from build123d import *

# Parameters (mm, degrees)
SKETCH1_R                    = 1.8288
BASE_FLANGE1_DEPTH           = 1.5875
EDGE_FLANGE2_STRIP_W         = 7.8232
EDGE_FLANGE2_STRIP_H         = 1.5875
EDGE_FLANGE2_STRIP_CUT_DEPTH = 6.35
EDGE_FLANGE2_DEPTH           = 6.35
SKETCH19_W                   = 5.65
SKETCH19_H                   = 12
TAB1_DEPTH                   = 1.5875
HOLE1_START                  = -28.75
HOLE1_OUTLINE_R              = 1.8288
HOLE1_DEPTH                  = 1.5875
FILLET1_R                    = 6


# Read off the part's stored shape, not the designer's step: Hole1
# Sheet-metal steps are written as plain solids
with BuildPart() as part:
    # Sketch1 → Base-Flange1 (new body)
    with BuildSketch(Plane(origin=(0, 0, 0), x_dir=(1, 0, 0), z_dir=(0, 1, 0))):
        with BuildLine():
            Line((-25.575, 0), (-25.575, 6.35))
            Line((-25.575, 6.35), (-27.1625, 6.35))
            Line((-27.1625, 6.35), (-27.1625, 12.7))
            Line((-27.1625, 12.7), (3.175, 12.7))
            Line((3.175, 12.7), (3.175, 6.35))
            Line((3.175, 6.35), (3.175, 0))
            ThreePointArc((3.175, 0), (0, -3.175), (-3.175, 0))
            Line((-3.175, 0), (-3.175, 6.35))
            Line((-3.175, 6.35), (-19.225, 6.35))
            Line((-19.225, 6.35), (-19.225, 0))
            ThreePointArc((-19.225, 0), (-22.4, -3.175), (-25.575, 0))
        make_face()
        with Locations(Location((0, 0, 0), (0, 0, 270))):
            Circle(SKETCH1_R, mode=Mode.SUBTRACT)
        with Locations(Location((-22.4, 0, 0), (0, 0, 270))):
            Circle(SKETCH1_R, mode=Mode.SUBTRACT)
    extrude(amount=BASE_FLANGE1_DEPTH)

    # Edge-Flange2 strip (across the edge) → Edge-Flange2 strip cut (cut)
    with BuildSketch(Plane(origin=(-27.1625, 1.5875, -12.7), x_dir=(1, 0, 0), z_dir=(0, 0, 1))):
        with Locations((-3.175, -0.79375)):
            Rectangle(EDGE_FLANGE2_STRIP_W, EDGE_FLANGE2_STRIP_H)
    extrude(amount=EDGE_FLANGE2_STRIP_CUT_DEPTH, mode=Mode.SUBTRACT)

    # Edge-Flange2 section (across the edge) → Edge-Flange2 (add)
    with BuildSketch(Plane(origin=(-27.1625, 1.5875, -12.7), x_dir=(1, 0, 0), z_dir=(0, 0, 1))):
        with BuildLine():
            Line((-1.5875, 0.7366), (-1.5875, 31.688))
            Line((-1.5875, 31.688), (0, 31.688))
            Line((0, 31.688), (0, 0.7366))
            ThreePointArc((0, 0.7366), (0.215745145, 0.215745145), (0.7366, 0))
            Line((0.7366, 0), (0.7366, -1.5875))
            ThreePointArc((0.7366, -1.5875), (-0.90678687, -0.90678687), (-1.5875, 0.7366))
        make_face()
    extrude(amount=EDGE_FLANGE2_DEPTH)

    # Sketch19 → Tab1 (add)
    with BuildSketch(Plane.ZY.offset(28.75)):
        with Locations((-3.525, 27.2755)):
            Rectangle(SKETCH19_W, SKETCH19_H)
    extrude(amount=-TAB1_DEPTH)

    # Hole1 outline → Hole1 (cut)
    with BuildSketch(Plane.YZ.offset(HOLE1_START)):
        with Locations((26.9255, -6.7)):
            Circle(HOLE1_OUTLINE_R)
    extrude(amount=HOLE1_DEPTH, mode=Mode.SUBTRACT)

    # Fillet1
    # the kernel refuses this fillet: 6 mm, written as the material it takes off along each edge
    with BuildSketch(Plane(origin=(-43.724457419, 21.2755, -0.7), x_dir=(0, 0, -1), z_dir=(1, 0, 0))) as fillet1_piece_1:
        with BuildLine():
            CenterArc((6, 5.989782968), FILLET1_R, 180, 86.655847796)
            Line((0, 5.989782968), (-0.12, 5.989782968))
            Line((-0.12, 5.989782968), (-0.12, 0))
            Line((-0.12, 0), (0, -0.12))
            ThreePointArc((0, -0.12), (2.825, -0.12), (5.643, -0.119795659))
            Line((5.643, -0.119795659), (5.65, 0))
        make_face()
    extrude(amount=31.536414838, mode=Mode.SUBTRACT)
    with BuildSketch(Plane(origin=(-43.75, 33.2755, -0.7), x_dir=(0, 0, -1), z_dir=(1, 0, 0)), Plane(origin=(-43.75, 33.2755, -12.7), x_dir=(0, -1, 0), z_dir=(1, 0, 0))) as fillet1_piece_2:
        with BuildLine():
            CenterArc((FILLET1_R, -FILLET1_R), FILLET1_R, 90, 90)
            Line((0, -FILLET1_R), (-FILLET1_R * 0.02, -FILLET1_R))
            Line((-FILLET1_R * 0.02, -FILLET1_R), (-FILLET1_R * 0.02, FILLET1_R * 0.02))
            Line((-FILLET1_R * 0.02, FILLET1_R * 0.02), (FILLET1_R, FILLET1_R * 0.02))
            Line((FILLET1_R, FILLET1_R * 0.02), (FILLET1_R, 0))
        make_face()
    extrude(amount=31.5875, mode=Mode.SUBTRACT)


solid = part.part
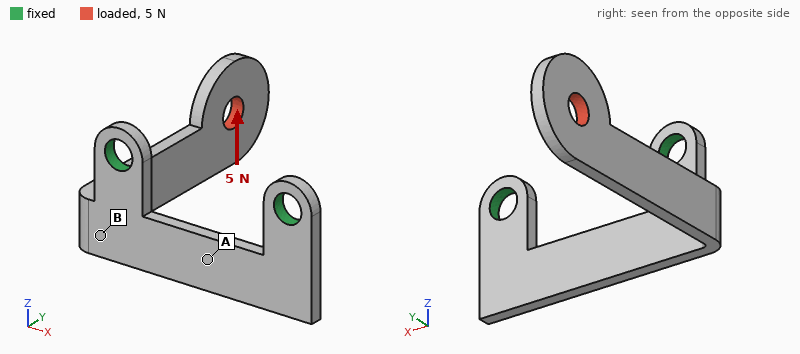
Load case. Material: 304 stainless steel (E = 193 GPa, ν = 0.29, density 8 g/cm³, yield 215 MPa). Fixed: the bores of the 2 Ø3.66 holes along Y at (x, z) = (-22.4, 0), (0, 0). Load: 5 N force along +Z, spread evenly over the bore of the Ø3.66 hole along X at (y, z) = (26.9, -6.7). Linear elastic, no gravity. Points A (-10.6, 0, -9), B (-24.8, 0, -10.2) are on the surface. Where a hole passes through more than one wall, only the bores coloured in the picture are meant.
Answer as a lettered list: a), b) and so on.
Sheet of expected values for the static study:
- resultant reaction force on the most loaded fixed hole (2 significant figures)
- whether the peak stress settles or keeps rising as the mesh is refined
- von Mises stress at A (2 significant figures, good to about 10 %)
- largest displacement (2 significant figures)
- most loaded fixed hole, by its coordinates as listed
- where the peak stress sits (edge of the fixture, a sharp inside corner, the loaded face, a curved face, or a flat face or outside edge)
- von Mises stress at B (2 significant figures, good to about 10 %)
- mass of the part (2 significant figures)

a) 6.0 N
b) keeps rising
c) 11 MPa
d) 87 µm
e) (-22.4, 0)
f) a sharp inside corner
g) 31 MPa
h) 6.7 g
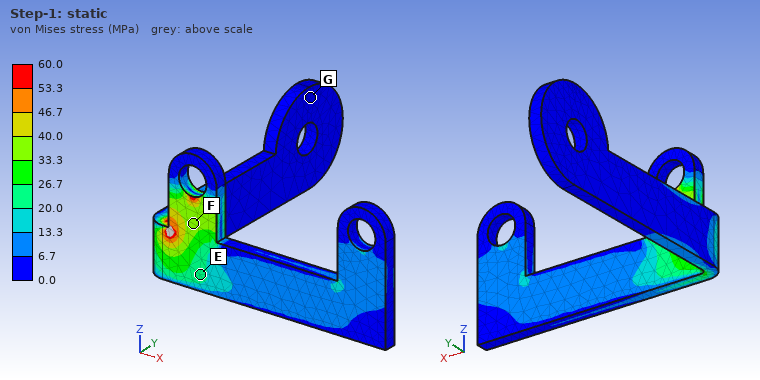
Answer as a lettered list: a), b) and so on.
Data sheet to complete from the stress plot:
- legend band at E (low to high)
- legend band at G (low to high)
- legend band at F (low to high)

a) 20.0 to 26.7 MPa
b) 0.0 to 6.7 MPa
c) 33.3 to 40.0 MPa
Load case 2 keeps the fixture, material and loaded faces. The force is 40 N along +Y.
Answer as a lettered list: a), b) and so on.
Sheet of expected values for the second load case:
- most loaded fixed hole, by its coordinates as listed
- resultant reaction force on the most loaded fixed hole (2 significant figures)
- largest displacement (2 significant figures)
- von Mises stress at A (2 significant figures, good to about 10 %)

a) (-22.4, 0)
b) 43 N
c) 85 µm
d) 12 MPa
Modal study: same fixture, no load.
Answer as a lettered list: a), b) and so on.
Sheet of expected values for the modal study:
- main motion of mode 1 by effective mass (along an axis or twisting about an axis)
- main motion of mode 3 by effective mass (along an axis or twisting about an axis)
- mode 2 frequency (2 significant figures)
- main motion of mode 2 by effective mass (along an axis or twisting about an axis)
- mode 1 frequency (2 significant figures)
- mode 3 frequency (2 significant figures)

a) along X
b) along Y
c) 1000 Hz
d) along Z
e) 760 Hz
f) 4600 Hz
